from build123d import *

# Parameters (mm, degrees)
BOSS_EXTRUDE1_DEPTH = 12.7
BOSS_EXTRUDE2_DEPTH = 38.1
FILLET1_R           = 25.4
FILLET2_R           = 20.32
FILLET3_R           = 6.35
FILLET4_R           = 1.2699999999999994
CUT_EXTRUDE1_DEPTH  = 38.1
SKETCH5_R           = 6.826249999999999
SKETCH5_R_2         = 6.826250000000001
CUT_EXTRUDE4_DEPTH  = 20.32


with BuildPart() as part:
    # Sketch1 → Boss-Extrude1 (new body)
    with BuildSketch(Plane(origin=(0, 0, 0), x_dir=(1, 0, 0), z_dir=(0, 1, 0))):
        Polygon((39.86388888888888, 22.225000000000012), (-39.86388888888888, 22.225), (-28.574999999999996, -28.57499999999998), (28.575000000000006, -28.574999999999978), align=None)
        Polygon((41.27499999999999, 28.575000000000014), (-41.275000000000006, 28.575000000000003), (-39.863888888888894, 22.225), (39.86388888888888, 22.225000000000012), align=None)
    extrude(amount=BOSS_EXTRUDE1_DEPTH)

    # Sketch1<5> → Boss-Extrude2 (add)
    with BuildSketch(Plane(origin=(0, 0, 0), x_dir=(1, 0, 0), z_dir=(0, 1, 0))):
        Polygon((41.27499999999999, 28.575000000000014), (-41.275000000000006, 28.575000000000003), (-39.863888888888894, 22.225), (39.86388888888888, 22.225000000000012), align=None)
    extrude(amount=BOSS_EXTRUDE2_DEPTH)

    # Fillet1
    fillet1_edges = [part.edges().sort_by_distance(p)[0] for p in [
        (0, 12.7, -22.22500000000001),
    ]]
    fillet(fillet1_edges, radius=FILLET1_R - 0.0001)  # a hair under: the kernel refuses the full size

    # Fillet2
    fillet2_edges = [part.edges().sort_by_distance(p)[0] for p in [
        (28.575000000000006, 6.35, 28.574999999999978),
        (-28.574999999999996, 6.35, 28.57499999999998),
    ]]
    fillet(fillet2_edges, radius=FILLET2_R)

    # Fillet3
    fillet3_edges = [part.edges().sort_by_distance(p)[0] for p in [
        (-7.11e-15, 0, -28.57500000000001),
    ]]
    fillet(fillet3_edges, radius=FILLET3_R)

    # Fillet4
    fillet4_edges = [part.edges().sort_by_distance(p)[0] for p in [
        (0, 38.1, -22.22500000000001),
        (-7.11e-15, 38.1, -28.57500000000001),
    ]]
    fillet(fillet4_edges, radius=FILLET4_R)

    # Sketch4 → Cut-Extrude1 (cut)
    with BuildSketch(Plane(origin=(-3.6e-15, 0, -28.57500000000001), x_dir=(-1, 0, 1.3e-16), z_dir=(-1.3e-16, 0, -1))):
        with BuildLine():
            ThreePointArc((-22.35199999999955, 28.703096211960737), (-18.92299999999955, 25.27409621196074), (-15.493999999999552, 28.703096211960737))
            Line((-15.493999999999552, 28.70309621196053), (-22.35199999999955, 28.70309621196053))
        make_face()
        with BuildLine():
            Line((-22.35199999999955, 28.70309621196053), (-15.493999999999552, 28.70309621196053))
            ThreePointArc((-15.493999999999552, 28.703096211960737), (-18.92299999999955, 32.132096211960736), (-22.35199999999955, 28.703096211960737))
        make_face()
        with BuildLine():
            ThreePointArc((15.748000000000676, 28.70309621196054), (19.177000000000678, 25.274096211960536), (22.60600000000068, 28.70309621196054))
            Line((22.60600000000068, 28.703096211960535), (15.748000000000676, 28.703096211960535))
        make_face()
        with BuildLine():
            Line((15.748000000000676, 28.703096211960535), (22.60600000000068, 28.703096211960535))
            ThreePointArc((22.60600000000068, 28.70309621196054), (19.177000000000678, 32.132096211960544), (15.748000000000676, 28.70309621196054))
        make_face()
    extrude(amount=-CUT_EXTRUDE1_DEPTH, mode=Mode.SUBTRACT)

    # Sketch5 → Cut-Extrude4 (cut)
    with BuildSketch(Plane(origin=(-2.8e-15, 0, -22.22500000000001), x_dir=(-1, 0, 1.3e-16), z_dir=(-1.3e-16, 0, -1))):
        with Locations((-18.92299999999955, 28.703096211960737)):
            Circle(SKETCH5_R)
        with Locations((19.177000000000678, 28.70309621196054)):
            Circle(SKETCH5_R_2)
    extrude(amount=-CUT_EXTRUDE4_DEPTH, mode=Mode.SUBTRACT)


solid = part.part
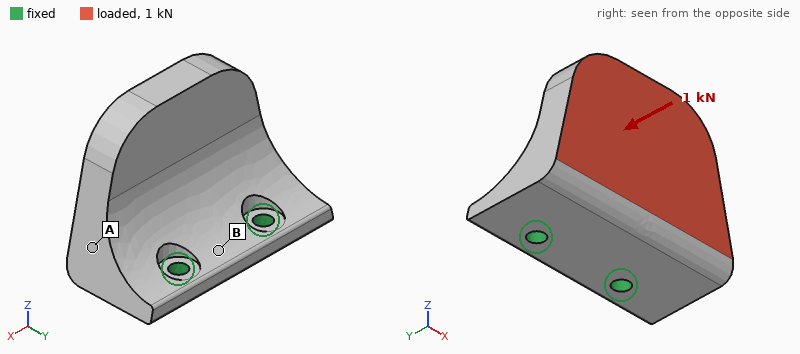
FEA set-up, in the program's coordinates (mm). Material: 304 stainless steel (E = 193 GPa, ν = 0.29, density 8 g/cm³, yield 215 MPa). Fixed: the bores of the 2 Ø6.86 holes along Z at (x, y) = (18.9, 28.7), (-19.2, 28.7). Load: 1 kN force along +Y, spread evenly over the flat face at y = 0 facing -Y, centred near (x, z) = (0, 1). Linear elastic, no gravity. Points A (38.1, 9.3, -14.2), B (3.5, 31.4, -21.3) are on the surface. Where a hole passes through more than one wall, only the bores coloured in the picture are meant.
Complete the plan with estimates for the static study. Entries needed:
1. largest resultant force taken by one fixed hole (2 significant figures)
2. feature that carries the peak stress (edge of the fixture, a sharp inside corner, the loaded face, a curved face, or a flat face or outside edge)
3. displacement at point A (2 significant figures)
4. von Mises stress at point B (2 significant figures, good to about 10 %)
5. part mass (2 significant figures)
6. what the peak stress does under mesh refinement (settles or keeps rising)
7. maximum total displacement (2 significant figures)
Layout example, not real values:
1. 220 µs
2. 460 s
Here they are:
1. 510 N
2. edge of the fixture
3. 11 µm
4. 13 MPa
5. 570 g
6. keeps rising
7. 36 µm
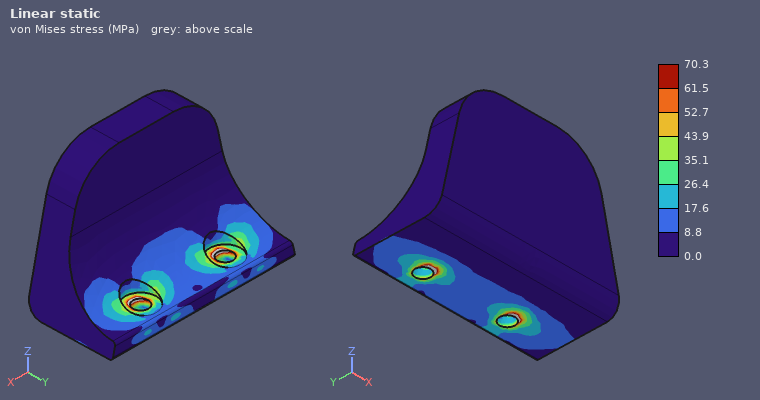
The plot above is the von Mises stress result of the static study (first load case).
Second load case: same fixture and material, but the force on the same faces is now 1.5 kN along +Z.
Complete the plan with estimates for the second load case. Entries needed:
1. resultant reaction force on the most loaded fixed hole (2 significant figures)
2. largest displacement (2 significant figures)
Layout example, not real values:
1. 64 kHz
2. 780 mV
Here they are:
1. 750 N
2. 50 µm
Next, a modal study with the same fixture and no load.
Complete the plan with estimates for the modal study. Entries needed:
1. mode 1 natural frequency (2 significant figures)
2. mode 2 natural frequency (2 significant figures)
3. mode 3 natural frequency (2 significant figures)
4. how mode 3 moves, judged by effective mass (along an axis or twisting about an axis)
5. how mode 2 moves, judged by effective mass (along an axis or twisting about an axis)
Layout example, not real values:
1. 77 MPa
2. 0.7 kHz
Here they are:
1. 1600 Hz
2. 4100 Hz
3. 7200 Hz
4. along X
5. along X
